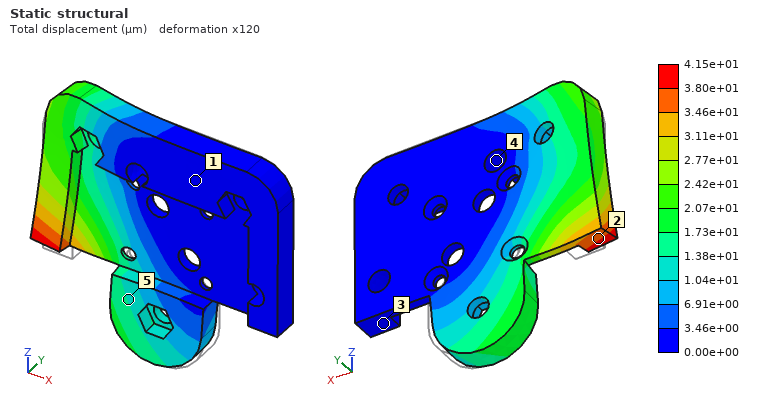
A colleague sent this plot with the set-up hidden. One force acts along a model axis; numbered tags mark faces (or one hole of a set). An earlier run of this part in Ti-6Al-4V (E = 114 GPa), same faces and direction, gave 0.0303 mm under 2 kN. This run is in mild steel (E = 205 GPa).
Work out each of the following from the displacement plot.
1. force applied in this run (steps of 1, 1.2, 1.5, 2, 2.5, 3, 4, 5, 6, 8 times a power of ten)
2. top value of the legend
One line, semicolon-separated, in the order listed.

5 kN; 4.15e+01 µm
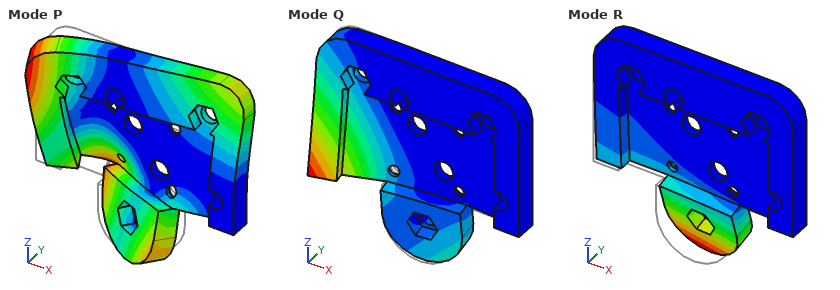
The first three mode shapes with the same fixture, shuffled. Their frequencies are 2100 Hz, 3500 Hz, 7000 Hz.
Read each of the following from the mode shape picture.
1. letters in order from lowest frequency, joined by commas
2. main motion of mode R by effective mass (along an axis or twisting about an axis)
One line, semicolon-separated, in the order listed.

R, Q, P; along Y
